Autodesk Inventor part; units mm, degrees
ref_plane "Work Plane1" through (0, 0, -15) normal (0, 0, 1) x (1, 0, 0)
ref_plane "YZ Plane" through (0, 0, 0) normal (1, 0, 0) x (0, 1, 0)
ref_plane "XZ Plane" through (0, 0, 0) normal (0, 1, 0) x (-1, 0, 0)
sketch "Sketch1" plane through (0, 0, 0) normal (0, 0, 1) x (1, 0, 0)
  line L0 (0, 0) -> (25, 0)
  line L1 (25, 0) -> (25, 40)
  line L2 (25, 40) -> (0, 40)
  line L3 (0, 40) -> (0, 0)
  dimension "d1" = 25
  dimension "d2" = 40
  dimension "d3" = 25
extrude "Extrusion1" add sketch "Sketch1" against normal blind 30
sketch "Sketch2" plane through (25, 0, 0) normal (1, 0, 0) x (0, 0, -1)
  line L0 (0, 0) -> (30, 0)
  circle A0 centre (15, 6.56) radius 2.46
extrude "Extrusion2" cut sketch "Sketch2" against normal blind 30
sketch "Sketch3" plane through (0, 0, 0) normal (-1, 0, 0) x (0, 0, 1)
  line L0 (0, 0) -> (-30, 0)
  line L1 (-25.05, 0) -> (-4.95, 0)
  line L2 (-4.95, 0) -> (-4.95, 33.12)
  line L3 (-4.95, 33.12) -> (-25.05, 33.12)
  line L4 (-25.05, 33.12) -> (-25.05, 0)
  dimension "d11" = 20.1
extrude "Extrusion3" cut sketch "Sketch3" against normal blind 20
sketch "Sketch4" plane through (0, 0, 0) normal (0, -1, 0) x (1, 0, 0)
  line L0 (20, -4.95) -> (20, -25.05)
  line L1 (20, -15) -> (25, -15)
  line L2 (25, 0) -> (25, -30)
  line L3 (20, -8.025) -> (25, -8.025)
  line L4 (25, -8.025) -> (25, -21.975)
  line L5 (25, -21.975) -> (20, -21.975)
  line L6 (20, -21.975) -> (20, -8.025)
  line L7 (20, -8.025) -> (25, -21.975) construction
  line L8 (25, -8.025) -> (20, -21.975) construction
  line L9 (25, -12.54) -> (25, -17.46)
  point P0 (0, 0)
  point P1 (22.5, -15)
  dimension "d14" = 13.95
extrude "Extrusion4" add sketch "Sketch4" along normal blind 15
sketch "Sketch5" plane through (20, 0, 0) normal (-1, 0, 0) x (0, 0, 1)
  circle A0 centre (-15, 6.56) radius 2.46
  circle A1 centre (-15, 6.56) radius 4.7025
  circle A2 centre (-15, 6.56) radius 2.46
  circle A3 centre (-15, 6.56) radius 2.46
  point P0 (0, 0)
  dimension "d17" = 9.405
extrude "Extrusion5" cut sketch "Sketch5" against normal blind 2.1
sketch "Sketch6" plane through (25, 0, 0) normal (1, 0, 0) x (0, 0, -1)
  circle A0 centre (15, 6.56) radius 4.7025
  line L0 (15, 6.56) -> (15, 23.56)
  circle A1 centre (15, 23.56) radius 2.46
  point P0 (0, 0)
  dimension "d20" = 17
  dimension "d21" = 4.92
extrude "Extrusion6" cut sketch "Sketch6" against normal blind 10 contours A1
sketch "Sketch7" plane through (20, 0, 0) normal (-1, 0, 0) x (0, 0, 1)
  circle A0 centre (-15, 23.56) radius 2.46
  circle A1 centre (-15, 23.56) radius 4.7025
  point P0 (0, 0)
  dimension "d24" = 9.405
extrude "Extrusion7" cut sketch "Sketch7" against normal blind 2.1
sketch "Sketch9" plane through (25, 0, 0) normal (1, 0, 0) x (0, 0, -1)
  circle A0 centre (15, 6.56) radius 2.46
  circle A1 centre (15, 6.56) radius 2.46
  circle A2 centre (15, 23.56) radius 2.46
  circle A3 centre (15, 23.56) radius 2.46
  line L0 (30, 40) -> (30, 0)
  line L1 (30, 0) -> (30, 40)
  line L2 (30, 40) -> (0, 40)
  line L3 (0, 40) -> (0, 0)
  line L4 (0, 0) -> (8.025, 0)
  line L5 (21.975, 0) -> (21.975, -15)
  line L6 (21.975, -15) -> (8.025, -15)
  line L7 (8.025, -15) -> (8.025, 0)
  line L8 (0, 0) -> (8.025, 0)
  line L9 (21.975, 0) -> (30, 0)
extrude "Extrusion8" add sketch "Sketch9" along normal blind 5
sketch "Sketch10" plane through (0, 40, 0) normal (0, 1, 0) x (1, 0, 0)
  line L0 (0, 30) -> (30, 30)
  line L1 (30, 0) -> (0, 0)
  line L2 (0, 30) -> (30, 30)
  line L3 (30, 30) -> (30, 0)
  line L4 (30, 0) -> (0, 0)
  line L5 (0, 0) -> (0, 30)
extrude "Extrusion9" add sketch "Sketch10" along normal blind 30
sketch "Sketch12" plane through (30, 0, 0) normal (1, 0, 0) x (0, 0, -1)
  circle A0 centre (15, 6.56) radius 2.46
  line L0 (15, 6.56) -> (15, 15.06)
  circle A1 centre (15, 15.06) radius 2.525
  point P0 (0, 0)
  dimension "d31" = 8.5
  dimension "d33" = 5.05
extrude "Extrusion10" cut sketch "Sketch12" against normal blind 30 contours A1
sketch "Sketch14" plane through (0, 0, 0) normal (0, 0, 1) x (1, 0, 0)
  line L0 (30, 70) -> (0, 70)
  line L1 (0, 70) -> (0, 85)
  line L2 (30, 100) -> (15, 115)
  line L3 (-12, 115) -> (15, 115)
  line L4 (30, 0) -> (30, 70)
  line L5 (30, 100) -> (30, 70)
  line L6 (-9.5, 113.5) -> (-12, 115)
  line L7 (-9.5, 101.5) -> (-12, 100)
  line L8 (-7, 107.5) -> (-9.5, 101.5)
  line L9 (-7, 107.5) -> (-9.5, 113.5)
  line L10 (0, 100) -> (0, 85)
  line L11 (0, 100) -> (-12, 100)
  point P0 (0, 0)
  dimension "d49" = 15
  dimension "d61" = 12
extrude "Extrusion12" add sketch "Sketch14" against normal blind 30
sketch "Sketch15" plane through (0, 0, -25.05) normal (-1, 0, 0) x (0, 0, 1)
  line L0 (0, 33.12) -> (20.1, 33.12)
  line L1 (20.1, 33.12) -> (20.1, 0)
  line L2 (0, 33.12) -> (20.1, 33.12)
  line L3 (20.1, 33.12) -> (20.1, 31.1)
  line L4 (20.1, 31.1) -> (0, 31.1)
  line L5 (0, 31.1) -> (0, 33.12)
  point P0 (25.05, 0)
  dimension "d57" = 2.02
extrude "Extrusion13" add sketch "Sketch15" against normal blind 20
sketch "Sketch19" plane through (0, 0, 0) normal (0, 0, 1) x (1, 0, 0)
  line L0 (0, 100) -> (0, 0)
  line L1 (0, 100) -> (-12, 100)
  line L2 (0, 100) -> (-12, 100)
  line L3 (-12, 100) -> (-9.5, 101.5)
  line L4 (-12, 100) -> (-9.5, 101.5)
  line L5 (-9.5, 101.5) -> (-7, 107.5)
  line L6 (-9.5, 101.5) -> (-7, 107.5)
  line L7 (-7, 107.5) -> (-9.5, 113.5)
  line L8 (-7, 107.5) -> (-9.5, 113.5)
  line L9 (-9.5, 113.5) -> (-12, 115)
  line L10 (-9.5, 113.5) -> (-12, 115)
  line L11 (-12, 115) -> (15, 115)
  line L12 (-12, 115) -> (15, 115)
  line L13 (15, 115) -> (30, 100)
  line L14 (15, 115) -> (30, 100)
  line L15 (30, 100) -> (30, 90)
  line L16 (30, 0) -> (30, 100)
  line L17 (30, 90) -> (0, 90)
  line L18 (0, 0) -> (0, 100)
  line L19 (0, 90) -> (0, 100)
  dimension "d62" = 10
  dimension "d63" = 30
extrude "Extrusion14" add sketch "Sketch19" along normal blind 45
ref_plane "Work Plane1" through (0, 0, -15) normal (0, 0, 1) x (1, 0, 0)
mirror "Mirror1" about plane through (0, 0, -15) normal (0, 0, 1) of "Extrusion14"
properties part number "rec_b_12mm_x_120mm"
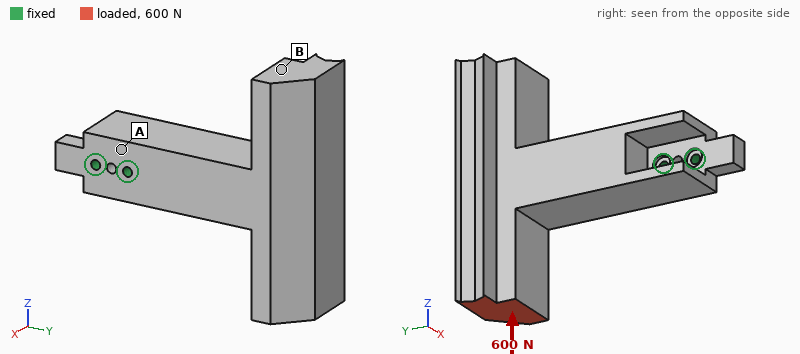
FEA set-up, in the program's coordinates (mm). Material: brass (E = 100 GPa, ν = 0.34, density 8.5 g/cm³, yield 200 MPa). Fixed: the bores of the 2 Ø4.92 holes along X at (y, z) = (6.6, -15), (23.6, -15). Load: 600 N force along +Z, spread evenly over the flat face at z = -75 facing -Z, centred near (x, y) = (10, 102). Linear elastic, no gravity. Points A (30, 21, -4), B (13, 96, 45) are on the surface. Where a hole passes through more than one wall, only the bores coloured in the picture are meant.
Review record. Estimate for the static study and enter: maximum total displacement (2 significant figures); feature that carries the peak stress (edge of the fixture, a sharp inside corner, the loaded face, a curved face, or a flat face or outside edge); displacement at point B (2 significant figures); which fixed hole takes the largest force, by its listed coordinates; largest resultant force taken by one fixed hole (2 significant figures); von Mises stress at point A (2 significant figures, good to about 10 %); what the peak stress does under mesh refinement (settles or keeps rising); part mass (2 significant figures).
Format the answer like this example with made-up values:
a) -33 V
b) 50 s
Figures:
a) 79 µm
b) edge of the fixture
c) 64 µm
d) (23.6, -15)
e) 2.6 kN
f) 16 MPa
g) keeps rising
h) 1.4 kg
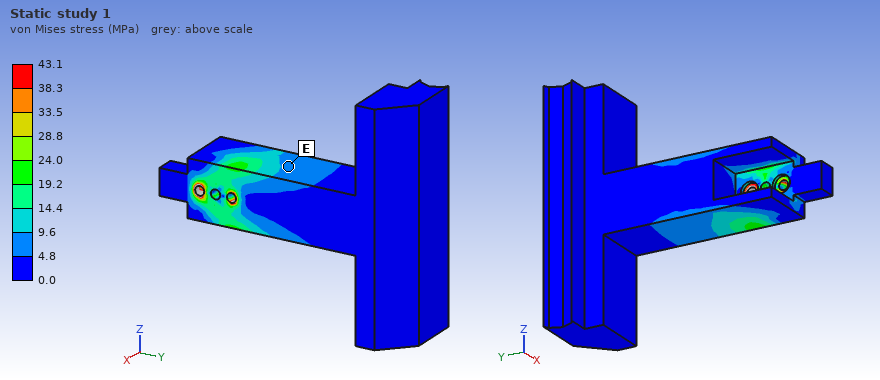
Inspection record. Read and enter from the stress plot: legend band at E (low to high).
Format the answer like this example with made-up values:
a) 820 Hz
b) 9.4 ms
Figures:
a) 4.8 to 9.6 MPa
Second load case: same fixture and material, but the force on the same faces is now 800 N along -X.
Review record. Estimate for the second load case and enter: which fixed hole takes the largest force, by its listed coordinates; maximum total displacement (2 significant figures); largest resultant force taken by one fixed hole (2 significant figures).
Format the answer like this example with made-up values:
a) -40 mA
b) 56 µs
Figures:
a) (23.6, -15)
b) 0.27 mm
c) 3.3 kN
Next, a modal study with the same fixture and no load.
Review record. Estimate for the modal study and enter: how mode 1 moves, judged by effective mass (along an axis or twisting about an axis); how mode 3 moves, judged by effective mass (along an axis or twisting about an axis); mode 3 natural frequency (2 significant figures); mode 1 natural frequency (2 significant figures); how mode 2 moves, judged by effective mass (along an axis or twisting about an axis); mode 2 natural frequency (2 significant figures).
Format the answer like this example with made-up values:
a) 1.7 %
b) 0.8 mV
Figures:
a) along X
b) twisting about Y
c) 700 Hz
d) 480 Hz
e) along Z
f) 510 Hz
